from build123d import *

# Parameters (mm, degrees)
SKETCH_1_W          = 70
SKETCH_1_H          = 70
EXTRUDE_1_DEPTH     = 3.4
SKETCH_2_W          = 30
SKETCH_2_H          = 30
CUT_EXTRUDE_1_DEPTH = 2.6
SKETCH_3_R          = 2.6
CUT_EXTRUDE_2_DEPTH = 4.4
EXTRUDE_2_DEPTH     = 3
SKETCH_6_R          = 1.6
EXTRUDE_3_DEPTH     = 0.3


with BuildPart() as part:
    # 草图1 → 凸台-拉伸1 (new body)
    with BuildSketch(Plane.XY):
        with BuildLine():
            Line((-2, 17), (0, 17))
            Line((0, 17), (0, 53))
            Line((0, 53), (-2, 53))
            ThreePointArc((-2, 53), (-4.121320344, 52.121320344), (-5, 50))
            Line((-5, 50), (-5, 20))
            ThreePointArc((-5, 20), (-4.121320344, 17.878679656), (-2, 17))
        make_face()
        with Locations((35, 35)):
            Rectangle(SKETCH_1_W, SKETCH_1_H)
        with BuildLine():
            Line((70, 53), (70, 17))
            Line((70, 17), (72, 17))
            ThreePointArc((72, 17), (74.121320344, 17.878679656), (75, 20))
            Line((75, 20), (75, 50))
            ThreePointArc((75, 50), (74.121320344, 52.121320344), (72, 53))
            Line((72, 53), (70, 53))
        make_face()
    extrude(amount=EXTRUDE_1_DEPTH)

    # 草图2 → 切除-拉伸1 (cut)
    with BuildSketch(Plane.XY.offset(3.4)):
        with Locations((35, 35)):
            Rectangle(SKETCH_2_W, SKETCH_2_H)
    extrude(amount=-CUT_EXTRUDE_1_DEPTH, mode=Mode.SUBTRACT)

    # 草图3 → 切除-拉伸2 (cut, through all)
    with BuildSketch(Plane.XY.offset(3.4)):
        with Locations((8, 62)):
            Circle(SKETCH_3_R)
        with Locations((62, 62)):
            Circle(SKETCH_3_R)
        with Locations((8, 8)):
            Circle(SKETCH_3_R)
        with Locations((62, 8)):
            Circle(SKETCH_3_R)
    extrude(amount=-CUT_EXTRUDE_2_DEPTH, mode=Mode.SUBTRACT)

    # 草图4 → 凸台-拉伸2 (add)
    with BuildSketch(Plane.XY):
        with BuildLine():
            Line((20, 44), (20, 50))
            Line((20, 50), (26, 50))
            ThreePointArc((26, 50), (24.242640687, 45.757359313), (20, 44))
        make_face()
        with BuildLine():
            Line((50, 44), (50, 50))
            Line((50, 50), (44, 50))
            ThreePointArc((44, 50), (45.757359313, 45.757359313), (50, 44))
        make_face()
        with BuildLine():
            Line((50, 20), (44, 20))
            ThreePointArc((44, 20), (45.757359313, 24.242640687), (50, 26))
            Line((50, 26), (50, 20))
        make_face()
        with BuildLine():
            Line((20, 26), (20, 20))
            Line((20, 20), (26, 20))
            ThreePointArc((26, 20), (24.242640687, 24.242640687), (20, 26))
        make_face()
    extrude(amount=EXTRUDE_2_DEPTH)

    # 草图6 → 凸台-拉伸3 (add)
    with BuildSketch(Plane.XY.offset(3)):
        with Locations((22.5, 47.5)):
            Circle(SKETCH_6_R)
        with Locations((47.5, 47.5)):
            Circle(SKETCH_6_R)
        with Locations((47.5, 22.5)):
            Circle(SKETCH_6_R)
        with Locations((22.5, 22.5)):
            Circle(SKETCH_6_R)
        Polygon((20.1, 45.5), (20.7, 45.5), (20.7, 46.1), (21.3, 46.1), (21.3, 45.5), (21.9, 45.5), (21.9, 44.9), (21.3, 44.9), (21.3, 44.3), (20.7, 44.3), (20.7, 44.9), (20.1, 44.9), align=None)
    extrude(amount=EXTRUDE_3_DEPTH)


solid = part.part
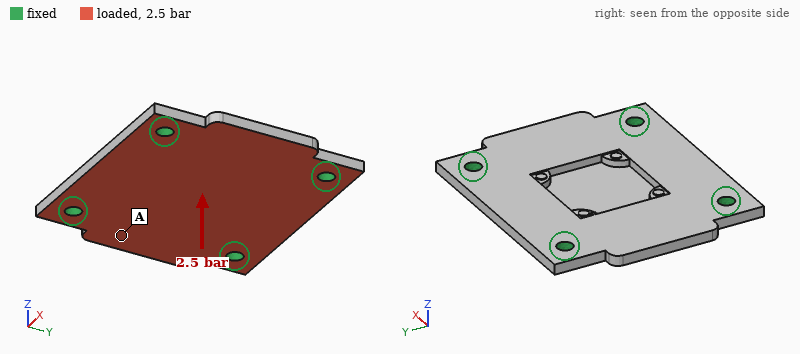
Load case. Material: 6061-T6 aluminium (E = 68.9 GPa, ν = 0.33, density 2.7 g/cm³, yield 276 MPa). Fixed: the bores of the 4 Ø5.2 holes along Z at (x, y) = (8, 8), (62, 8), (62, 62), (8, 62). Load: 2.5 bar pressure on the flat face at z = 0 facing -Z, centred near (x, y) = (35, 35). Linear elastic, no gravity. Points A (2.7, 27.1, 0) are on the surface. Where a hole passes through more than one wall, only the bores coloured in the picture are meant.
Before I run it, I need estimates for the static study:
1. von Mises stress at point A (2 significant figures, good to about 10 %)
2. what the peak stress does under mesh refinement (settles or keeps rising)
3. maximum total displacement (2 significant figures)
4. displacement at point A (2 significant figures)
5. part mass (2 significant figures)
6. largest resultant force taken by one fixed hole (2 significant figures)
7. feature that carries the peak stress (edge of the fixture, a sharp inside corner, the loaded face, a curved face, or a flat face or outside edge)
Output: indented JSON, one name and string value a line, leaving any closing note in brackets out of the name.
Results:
{
  "von Mises stress at point A": "14 MPa",
  "what the peak stress does under mesh refinement": "keeps rising",
  "maximum total displacement": "0.14 mm",
  "displacement at point A": "0.023 mm",
  "part mass": "42 g",
  "largest resultant force taken by one fixed hole": "350 N",
  "feature that carries the peak stress": "edge of the fixture"
}
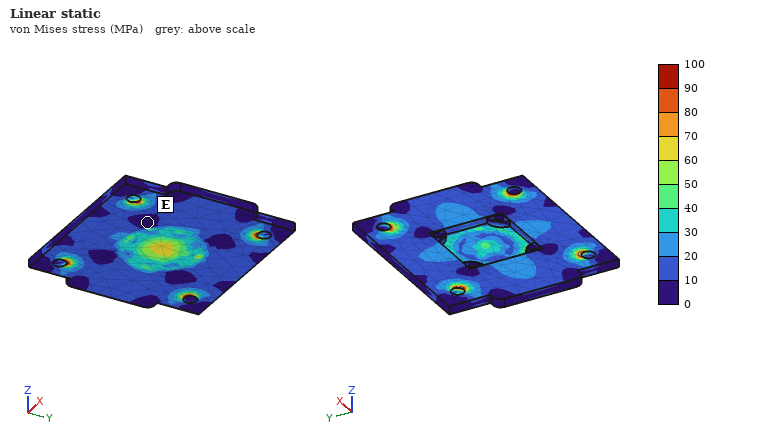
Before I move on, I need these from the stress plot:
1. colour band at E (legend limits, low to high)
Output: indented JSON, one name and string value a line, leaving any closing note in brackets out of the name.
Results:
{
  "colour band at E": "0 to 10 MPa"
}
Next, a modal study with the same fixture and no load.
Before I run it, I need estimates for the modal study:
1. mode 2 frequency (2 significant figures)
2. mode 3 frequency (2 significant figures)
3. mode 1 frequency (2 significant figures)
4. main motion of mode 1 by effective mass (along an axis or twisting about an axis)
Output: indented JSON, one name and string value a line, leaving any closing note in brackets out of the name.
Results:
{
  "mode 2 frequency": "6000 Hz",
  "mode 3 frequency": "6000 Hz",
  "mode 1 frequency": "5000 Hz",
  "main motion of mode 1 by effective mass": "along Z"
}
